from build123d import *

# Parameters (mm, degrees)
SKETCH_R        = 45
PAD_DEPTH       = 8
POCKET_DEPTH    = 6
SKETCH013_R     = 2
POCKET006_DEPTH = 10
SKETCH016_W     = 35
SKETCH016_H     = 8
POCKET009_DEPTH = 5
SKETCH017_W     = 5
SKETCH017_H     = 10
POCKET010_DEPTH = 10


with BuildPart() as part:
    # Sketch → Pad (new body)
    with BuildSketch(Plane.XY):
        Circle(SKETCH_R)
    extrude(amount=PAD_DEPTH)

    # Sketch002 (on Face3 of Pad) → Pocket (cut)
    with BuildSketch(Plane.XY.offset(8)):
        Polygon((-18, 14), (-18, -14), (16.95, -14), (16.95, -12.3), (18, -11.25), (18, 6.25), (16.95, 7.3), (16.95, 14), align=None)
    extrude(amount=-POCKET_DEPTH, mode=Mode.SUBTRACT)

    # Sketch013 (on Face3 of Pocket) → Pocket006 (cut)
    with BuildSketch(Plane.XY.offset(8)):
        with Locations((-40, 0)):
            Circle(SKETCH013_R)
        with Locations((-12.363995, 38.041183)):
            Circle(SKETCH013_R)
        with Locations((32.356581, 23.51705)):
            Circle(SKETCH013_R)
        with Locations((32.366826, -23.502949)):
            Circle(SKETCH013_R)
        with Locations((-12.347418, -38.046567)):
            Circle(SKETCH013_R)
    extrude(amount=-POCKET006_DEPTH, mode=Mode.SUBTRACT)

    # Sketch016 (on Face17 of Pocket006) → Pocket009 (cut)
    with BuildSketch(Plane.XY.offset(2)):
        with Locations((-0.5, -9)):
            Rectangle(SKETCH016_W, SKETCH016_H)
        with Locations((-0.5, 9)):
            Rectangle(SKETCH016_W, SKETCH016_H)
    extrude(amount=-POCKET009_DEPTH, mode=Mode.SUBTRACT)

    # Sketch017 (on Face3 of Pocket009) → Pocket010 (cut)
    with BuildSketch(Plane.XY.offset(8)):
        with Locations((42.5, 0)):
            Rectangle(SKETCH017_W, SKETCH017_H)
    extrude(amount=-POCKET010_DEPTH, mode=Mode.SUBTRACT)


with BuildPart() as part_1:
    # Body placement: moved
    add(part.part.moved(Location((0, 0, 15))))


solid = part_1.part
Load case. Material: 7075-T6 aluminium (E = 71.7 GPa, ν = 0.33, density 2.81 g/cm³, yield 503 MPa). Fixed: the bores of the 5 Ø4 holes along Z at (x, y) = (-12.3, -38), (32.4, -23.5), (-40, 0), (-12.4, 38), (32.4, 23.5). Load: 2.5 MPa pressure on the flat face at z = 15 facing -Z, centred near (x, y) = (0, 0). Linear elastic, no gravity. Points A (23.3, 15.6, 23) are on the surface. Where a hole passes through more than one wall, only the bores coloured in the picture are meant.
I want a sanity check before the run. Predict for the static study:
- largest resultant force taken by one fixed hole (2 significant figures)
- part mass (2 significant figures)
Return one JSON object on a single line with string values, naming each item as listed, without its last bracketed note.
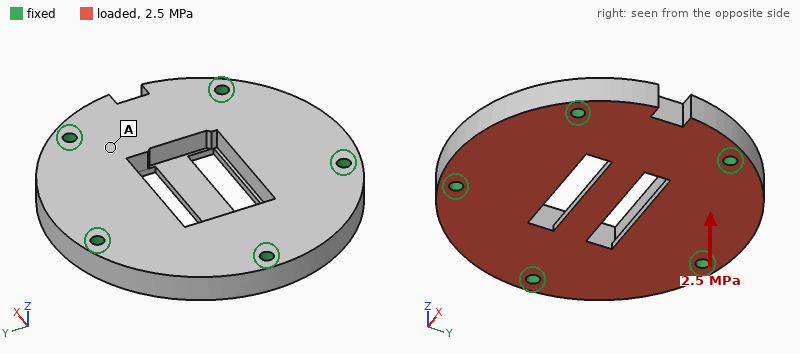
{"largest resultant force taken by one fixed hole": "3.0 kN", "part mass": "120 g"}
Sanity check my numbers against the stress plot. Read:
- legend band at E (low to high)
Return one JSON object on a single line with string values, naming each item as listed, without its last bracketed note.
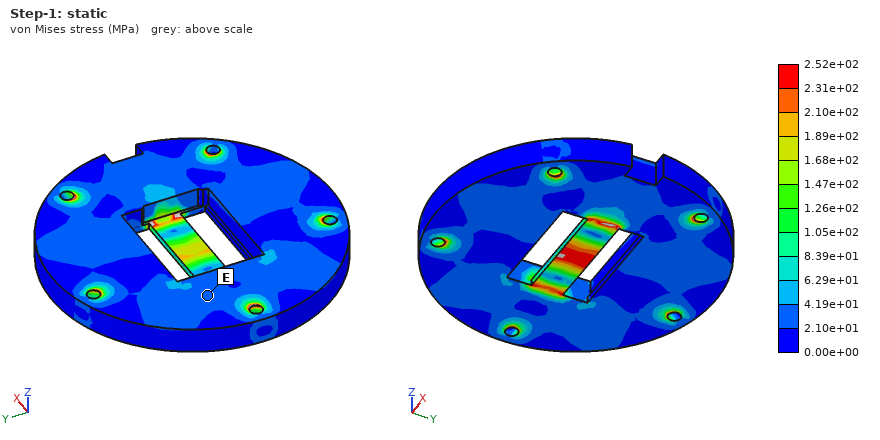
{"legend band at E": "2.10e+01 to 4.19e+01 MPa"}
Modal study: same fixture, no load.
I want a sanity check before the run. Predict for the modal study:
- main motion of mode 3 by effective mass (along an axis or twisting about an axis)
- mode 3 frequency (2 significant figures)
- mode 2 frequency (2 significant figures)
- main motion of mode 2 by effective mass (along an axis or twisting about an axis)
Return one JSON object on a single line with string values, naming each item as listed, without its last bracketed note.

{"main motion of mode 3 by effective mass": "twisting about X", "mode 3 frequency": "13 kHz", "mode 2 frequency": "11 kHz", "main motion of mode 2 by effective mass": "along Z"}
